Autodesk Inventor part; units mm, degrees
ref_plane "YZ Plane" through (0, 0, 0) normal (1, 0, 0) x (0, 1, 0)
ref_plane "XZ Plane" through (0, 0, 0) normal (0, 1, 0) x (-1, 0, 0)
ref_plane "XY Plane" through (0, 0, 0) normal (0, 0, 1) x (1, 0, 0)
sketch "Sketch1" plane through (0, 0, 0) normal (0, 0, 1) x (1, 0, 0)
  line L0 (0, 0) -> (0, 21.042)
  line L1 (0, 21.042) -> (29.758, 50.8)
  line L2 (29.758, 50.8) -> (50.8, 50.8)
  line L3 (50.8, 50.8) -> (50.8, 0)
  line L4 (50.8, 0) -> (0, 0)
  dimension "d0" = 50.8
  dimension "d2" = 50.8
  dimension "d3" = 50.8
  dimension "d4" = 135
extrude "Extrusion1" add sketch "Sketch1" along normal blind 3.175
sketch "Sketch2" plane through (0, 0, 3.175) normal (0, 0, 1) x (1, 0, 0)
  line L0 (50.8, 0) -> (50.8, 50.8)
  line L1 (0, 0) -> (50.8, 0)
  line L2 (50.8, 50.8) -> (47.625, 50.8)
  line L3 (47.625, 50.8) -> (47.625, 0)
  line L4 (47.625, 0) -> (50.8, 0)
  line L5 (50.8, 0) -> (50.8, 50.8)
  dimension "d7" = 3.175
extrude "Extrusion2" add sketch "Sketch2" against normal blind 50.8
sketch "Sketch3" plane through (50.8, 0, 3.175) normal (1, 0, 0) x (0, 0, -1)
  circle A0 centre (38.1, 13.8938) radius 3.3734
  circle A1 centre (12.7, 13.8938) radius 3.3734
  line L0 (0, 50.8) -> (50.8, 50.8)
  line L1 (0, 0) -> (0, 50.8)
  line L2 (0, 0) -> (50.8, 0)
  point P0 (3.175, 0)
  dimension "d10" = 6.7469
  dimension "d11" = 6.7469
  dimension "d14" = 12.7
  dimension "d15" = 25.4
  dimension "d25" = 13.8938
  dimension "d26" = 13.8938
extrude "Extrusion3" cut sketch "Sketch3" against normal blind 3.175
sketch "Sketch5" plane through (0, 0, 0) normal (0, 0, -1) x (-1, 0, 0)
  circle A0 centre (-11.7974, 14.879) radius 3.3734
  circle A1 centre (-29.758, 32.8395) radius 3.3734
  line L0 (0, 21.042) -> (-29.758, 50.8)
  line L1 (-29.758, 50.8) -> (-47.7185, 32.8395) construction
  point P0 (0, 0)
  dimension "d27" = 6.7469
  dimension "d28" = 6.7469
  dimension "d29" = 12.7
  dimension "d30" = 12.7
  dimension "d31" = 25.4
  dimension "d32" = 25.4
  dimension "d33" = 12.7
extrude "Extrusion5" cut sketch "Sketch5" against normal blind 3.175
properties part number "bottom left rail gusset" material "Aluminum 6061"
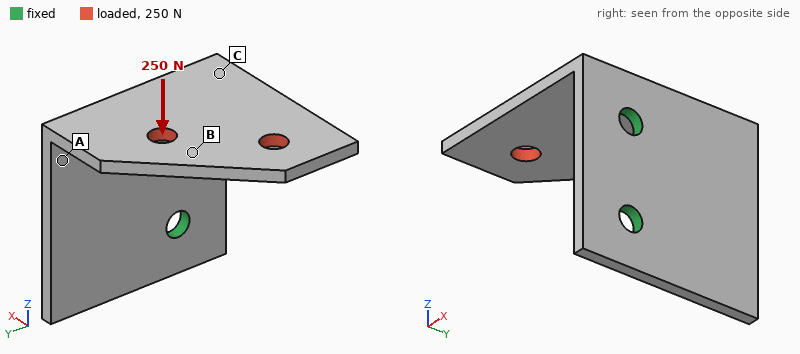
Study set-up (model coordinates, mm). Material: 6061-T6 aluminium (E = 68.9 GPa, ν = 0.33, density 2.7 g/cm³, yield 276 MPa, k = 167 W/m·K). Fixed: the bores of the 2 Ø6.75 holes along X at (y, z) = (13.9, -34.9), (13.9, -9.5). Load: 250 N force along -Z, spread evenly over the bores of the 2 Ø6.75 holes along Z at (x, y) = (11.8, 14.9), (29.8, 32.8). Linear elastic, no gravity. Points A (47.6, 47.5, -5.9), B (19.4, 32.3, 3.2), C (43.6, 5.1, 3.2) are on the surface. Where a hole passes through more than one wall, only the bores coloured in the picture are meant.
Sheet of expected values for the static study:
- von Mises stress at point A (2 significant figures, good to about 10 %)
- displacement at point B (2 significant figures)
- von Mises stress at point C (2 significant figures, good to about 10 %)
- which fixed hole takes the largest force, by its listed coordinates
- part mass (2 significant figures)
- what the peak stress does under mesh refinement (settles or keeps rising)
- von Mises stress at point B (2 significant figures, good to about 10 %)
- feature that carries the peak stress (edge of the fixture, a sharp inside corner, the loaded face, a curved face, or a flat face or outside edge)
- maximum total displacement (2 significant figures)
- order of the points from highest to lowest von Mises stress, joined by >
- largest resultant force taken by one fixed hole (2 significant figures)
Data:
48 MPa
0.48 mm
73 MPa
(13.9, -9.5)
38 g
keeps rising
22 MPa
edge of the fixture
0.89 mm
C > A > B
220 N
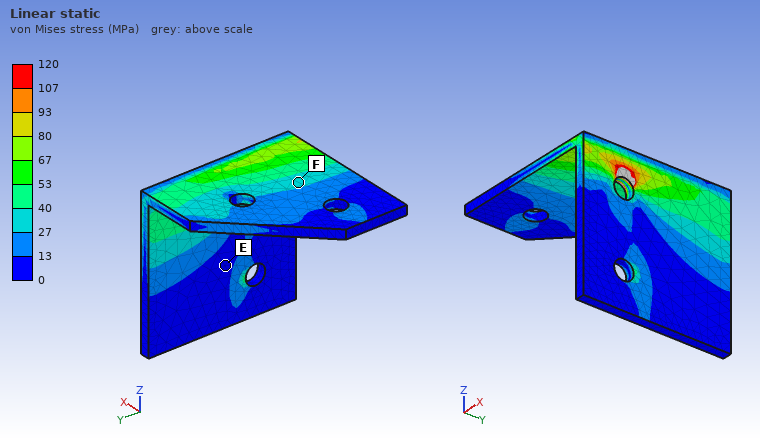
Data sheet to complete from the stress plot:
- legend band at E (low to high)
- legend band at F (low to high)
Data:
0 to 13 MPa
27 to 40 MPa
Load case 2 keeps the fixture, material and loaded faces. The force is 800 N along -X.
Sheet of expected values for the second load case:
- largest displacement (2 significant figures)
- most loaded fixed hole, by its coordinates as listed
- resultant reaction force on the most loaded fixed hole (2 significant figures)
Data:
0.42 mm
(13.9, -9.5)
870 N
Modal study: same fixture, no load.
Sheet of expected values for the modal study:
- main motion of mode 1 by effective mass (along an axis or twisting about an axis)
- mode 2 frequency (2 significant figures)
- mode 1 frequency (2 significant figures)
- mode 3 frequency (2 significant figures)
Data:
along Z
1500 Hz
980 Hz
2800 Hz
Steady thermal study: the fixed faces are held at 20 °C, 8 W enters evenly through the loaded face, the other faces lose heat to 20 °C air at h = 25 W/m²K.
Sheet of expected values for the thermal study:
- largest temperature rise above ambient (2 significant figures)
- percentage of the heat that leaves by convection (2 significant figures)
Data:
14 K
16 %
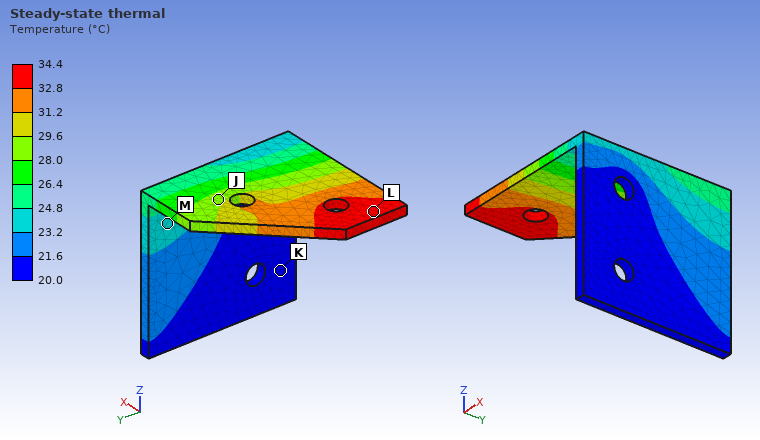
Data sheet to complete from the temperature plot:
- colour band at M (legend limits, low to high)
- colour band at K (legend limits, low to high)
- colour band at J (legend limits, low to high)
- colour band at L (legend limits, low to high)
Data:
23.2 to 24.8 °C
20.0 to 21.6 °C
28.0 to 29.6 °C
32.8 to 34.4 °C
